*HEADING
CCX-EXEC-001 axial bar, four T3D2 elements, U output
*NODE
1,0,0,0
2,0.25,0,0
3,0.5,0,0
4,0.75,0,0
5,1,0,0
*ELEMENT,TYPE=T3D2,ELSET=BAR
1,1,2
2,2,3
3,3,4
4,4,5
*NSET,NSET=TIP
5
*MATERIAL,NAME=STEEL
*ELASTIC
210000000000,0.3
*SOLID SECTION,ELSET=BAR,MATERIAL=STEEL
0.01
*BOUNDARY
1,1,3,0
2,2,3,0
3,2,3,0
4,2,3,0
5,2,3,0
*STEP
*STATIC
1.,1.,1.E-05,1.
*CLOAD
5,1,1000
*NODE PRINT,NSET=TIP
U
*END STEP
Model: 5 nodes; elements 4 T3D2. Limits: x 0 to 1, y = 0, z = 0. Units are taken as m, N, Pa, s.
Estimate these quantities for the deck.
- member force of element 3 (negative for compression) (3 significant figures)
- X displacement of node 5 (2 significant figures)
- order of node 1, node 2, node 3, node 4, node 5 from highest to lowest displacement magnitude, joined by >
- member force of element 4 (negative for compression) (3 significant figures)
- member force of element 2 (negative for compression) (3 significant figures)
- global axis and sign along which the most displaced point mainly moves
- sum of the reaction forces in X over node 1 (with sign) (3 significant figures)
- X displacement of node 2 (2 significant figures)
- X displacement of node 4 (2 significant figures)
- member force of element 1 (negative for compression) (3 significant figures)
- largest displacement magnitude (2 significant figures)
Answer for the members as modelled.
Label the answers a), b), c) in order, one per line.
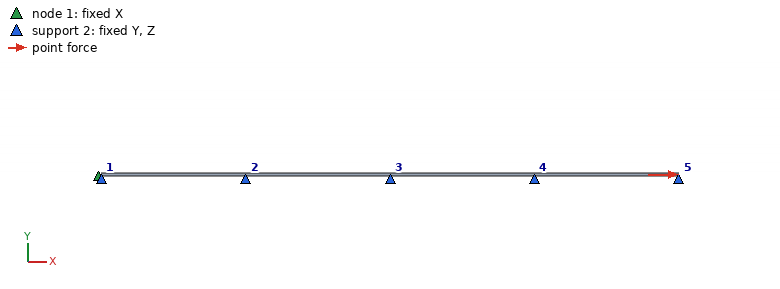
a) 1000 N
b) 4.8e-07 m
c) node 5 > node 4 > node 3 > node 2 > node 1
d) 1000 N
e) 1000 N
f) +X
g) -1000 N
h) 1.2e-07 m
i) 3.6e-07 m
j) 1000 N
k) 4.8e-07 m
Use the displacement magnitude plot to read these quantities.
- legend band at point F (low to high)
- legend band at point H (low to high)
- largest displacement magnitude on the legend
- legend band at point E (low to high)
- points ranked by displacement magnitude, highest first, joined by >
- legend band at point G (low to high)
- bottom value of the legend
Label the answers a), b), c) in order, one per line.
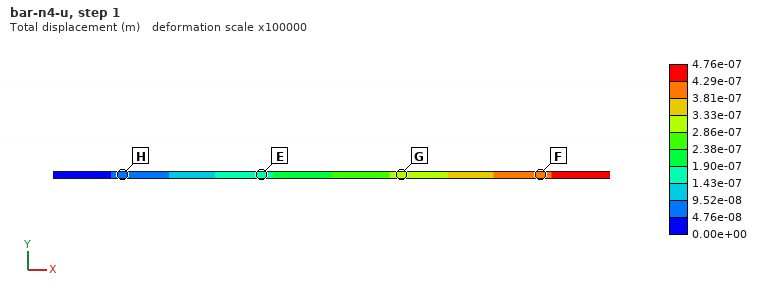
a) 3.81e-07 to 4.29e-07 m
b) 4.76e-08 to 9.52e-08 m
c) 4.76e-07 m
d) 1.43e-07 to 1.90e-07 m
e) F > G > E > H
f) 2.86e-07 to 3.33e-07 m
g) 0.00e+00 m
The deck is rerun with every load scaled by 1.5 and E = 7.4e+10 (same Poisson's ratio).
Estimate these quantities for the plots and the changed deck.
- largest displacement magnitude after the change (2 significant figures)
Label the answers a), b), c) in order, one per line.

a) 2.0e-06 m
